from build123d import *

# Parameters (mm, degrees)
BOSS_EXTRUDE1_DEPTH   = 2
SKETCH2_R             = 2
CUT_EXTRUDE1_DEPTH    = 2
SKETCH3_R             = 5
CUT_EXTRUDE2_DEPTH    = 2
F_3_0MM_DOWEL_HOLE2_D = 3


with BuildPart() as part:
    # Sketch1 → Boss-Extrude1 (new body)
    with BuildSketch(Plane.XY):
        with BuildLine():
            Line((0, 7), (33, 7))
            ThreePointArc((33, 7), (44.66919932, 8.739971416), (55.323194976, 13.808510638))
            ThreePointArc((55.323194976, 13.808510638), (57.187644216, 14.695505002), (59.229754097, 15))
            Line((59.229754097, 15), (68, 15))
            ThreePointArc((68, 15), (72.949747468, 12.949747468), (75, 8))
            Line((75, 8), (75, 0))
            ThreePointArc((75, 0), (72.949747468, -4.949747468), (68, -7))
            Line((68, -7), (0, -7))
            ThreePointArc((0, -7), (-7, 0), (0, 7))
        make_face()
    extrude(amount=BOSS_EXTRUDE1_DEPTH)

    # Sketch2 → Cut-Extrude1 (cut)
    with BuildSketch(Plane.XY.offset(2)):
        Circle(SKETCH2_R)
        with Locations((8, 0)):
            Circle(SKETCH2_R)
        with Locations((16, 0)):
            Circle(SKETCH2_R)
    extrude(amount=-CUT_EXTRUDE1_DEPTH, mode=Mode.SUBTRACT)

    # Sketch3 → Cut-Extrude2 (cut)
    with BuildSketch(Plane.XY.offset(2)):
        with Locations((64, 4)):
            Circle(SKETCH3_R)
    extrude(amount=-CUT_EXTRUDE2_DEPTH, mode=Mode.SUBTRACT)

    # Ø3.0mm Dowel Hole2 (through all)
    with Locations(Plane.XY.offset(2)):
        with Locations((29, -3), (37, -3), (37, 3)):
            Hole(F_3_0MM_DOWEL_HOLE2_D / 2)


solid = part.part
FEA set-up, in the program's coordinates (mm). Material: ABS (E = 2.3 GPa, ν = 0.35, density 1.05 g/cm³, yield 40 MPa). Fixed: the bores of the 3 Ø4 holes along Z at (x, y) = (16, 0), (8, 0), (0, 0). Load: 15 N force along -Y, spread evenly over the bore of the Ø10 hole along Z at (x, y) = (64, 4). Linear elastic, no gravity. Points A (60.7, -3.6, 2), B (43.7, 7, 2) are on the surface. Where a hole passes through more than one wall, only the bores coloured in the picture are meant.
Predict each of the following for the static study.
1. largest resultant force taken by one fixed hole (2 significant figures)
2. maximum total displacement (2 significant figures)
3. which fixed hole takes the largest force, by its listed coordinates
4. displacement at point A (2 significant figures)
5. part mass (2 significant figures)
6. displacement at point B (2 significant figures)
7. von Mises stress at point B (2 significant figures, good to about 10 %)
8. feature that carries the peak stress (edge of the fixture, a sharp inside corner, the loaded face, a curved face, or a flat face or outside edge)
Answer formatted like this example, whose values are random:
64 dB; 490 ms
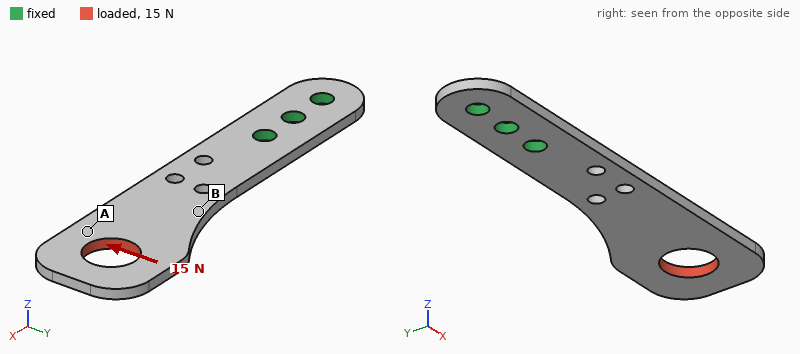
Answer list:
51 N; 0.95 mm; (16, 0); 0.66 mm; 2.5 g; 0.35 mm; 3.0 MPa; edge of the fixture
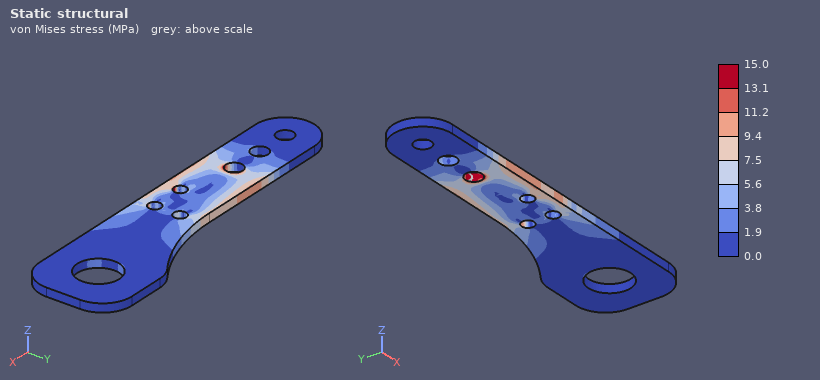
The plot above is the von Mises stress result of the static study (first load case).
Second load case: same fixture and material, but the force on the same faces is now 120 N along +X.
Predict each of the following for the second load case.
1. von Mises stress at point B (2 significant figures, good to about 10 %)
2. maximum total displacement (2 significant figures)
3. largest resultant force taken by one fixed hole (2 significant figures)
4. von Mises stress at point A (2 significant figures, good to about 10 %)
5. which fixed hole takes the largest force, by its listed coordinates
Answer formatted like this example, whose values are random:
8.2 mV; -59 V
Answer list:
8.4 MPa; 0.79 mm; 100 N; 3.3 MPa; (16, 0)
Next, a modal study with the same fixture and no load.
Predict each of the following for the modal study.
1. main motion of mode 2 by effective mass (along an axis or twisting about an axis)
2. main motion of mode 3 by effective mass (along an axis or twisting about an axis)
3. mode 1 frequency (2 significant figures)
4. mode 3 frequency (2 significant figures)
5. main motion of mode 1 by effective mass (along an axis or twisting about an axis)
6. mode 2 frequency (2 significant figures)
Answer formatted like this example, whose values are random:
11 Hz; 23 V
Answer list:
twisting about X; along Y; 130 Hz; 730 Hz; along Z; 640 Hz
